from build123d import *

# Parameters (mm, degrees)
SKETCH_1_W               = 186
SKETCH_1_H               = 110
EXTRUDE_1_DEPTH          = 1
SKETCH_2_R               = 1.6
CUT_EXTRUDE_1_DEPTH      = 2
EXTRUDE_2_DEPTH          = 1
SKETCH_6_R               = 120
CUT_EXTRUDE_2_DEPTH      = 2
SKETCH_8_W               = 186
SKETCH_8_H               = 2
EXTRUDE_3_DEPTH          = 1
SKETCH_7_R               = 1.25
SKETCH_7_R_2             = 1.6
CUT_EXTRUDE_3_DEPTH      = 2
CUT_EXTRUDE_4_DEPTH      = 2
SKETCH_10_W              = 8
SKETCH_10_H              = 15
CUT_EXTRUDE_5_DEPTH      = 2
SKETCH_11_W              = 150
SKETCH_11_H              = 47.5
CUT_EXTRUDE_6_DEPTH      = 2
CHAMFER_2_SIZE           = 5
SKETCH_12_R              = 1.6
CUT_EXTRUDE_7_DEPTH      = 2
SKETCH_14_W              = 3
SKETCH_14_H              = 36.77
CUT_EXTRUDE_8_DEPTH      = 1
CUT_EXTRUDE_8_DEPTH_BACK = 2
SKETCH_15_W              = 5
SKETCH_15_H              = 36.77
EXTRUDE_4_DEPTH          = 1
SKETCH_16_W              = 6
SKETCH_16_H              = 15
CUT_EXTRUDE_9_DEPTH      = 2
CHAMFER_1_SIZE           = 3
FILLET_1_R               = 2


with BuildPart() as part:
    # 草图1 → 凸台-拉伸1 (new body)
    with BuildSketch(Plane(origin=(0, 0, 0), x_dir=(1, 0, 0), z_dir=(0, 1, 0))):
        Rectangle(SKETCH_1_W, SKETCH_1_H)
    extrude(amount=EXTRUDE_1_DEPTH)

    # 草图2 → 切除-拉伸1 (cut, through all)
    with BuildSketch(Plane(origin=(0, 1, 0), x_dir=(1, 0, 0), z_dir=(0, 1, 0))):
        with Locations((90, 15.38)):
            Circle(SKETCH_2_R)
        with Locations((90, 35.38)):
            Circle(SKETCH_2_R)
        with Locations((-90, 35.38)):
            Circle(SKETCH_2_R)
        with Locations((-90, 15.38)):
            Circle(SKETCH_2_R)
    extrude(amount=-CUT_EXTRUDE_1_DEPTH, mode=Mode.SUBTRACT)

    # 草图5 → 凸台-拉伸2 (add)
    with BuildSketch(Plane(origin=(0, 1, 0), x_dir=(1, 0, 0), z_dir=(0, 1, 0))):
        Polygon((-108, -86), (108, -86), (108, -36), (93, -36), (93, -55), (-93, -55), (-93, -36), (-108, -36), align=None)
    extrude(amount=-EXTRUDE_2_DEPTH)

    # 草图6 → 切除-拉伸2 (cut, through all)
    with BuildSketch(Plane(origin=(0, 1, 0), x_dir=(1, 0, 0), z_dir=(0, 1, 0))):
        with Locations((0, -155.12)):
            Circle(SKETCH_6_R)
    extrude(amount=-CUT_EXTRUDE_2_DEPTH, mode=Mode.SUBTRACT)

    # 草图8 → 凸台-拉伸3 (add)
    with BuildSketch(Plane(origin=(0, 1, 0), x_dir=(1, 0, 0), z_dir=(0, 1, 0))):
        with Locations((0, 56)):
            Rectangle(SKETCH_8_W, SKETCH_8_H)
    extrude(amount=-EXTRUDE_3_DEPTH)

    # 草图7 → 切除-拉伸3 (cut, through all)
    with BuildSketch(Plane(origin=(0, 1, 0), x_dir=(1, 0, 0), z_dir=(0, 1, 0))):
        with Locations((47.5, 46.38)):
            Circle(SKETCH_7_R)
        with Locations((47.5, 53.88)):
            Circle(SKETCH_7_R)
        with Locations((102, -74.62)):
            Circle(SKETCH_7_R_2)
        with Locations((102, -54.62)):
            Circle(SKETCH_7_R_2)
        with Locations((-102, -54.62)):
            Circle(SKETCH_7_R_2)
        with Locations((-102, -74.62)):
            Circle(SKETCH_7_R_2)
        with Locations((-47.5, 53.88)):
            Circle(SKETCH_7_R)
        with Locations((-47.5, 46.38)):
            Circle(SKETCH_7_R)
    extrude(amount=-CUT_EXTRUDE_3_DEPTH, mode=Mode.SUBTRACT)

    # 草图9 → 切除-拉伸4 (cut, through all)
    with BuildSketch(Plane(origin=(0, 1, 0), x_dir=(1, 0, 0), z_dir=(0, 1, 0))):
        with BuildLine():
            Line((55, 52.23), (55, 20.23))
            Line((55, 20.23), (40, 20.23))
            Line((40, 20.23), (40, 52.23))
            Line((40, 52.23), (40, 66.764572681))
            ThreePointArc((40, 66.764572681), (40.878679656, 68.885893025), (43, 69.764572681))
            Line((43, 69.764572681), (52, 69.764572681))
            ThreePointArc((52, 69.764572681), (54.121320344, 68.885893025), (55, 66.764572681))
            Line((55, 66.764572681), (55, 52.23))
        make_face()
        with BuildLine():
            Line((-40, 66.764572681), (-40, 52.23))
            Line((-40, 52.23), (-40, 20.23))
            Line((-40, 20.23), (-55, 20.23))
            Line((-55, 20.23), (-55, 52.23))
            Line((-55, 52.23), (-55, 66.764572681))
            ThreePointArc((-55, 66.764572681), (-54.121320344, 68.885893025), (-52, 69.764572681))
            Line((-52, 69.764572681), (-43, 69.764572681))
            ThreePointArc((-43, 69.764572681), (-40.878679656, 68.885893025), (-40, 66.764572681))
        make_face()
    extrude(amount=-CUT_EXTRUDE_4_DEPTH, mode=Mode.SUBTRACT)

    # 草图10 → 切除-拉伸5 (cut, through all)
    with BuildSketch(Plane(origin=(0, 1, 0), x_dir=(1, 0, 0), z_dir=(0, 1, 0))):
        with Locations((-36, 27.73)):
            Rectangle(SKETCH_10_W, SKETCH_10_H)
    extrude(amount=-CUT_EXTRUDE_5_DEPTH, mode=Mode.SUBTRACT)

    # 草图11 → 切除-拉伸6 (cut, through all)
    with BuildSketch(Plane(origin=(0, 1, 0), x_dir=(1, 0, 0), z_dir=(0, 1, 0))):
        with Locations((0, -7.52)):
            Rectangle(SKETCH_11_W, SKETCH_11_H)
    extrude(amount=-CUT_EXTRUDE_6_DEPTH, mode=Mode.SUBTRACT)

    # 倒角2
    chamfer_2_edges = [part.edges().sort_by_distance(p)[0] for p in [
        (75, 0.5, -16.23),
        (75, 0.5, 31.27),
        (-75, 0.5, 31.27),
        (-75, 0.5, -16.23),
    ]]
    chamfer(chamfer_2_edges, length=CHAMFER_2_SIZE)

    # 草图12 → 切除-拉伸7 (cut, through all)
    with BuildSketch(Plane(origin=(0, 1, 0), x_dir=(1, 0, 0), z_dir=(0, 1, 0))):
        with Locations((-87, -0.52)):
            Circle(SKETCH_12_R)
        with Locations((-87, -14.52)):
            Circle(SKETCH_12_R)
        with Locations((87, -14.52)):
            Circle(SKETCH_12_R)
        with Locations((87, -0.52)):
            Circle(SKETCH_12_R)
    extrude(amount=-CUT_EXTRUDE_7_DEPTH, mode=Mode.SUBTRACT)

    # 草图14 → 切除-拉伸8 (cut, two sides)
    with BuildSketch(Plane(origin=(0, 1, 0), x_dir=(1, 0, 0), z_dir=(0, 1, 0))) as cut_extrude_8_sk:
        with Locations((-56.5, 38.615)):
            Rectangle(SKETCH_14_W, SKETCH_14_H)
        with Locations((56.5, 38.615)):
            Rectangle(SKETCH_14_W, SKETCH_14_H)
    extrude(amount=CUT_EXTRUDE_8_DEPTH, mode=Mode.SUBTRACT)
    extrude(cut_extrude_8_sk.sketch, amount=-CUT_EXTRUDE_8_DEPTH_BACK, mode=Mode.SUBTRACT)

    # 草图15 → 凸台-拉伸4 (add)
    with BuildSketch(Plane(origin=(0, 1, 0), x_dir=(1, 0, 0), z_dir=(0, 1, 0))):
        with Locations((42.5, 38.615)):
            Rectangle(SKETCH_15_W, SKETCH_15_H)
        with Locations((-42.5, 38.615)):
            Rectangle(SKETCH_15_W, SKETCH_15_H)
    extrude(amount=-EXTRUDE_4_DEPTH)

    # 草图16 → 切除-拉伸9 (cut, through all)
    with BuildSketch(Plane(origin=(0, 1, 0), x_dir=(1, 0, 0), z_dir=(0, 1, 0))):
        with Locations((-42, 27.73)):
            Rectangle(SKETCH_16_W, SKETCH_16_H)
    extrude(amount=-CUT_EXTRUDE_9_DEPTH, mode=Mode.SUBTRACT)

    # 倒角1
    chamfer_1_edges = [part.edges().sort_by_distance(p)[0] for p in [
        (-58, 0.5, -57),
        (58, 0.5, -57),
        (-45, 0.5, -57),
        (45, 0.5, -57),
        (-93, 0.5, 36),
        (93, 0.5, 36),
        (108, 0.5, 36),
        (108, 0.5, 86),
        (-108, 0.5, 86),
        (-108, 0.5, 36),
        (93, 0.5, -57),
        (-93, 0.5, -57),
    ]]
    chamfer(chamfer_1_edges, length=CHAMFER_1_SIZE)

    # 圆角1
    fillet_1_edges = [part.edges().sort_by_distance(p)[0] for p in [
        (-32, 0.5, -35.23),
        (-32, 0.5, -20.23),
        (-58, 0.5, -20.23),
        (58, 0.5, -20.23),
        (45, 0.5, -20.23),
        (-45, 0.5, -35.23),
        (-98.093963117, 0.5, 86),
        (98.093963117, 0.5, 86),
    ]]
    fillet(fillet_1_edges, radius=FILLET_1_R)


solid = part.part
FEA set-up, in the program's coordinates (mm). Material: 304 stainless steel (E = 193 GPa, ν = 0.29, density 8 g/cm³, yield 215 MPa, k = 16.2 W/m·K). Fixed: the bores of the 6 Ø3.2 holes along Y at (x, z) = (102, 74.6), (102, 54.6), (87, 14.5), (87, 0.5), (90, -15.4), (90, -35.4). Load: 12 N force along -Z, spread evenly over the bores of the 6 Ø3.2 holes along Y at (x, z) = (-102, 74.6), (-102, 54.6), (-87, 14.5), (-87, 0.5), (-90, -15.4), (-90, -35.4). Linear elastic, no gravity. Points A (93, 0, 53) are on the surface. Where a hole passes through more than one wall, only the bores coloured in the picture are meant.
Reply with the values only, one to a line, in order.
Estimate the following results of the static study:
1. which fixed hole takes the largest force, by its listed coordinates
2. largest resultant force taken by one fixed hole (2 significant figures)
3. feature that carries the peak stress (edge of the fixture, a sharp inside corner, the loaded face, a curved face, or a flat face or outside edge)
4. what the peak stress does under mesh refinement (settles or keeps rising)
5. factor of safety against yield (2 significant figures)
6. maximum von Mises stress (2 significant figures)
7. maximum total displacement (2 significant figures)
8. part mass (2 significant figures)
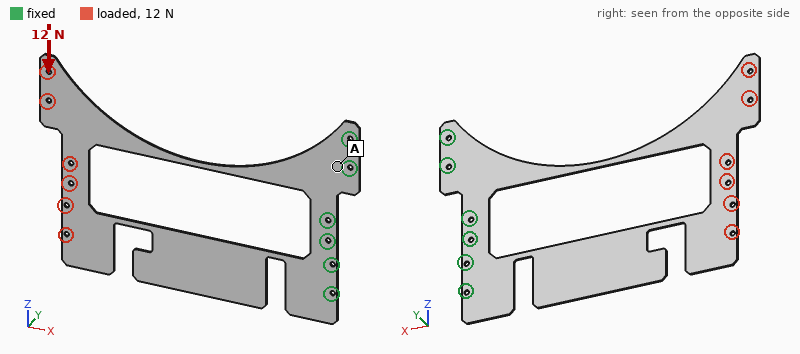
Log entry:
(102, 54.6)
16 N
a curved face
settles
3.7
57 MPa
0.15 mm
100 g
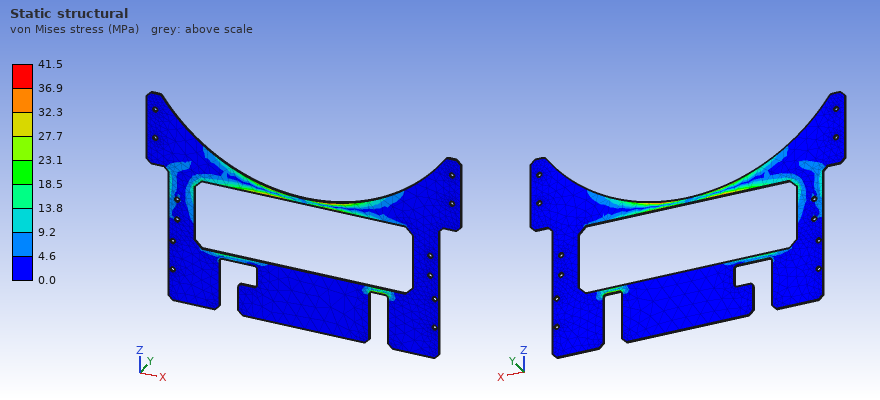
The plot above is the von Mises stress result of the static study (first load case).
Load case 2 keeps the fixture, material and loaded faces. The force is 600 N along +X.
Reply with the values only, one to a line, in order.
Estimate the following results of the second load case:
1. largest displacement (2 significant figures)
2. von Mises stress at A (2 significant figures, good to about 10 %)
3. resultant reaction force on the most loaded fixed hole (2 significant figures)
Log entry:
0.22 mm
15 MPa
240 N
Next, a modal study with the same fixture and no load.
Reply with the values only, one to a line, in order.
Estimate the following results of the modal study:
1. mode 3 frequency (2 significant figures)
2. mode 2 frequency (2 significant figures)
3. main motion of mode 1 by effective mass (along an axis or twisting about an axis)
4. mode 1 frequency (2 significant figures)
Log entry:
91 Hz
32 Hz
along Y
12 Hz
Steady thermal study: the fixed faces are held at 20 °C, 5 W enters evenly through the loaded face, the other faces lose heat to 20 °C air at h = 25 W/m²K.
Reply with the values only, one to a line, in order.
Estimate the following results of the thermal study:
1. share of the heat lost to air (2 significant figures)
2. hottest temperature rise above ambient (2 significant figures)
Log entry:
100 %
60 K
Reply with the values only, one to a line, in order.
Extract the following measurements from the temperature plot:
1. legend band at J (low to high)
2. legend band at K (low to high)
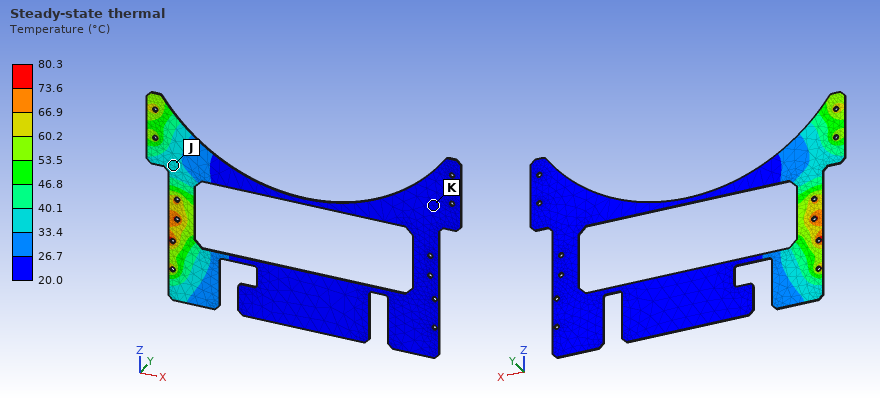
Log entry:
33.4 to 40.1 °C
20.0 to 26.7 °C
